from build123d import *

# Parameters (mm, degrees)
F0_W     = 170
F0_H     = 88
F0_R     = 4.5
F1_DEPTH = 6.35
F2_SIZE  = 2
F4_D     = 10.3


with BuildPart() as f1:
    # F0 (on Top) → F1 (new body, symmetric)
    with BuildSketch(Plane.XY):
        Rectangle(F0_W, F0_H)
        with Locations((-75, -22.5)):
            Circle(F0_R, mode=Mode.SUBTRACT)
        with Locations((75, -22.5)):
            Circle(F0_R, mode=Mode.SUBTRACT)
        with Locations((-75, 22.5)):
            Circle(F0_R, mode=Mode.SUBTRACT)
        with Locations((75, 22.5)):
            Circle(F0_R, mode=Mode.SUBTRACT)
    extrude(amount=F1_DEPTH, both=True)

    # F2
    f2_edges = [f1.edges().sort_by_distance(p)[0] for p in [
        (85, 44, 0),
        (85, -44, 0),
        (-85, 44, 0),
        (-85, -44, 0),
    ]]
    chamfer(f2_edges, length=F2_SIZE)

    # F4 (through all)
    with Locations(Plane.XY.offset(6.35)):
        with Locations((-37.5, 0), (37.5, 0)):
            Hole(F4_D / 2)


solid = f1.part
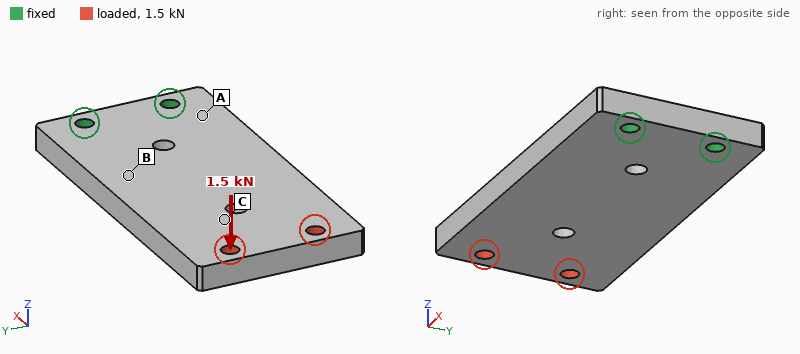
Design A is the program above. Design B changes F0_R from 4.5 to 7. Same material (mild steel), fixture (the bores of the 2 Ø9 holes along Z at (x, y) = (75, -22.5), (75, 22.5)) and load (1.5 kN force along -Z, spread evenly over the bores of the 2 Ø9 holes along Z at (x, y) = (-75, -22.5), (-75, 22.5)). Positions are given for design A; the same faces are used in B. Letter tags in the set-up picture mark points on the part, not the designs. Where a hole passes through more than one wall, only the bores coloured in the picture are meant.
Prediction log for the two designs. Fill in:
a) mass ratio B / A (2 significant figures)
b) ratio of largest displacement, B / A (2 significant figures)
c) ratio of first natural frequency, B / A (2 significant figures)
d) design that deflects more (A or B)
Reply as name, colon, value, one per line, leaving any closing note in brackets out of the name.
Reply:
mass ratio B / A: 0.98
ratio of largest displacement, B / A: 0.92
ratio of first natural frequency, B / A: 1.1
design that deflects more: A
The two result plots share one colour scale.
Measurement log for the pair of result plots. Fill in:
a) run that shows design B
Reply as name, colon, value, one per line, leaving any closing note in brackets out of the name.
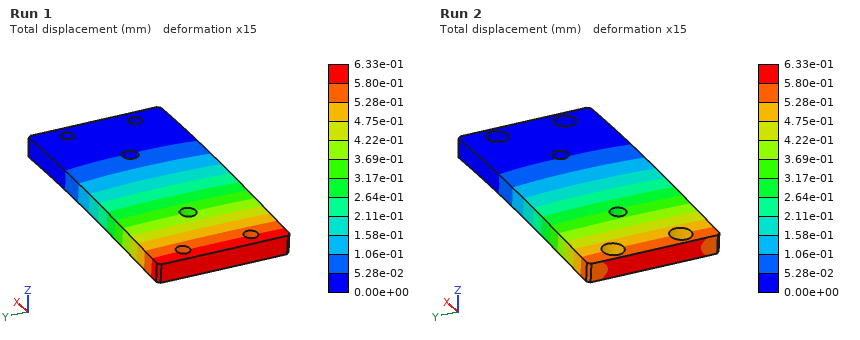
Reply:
run that shows design B: Run 2
